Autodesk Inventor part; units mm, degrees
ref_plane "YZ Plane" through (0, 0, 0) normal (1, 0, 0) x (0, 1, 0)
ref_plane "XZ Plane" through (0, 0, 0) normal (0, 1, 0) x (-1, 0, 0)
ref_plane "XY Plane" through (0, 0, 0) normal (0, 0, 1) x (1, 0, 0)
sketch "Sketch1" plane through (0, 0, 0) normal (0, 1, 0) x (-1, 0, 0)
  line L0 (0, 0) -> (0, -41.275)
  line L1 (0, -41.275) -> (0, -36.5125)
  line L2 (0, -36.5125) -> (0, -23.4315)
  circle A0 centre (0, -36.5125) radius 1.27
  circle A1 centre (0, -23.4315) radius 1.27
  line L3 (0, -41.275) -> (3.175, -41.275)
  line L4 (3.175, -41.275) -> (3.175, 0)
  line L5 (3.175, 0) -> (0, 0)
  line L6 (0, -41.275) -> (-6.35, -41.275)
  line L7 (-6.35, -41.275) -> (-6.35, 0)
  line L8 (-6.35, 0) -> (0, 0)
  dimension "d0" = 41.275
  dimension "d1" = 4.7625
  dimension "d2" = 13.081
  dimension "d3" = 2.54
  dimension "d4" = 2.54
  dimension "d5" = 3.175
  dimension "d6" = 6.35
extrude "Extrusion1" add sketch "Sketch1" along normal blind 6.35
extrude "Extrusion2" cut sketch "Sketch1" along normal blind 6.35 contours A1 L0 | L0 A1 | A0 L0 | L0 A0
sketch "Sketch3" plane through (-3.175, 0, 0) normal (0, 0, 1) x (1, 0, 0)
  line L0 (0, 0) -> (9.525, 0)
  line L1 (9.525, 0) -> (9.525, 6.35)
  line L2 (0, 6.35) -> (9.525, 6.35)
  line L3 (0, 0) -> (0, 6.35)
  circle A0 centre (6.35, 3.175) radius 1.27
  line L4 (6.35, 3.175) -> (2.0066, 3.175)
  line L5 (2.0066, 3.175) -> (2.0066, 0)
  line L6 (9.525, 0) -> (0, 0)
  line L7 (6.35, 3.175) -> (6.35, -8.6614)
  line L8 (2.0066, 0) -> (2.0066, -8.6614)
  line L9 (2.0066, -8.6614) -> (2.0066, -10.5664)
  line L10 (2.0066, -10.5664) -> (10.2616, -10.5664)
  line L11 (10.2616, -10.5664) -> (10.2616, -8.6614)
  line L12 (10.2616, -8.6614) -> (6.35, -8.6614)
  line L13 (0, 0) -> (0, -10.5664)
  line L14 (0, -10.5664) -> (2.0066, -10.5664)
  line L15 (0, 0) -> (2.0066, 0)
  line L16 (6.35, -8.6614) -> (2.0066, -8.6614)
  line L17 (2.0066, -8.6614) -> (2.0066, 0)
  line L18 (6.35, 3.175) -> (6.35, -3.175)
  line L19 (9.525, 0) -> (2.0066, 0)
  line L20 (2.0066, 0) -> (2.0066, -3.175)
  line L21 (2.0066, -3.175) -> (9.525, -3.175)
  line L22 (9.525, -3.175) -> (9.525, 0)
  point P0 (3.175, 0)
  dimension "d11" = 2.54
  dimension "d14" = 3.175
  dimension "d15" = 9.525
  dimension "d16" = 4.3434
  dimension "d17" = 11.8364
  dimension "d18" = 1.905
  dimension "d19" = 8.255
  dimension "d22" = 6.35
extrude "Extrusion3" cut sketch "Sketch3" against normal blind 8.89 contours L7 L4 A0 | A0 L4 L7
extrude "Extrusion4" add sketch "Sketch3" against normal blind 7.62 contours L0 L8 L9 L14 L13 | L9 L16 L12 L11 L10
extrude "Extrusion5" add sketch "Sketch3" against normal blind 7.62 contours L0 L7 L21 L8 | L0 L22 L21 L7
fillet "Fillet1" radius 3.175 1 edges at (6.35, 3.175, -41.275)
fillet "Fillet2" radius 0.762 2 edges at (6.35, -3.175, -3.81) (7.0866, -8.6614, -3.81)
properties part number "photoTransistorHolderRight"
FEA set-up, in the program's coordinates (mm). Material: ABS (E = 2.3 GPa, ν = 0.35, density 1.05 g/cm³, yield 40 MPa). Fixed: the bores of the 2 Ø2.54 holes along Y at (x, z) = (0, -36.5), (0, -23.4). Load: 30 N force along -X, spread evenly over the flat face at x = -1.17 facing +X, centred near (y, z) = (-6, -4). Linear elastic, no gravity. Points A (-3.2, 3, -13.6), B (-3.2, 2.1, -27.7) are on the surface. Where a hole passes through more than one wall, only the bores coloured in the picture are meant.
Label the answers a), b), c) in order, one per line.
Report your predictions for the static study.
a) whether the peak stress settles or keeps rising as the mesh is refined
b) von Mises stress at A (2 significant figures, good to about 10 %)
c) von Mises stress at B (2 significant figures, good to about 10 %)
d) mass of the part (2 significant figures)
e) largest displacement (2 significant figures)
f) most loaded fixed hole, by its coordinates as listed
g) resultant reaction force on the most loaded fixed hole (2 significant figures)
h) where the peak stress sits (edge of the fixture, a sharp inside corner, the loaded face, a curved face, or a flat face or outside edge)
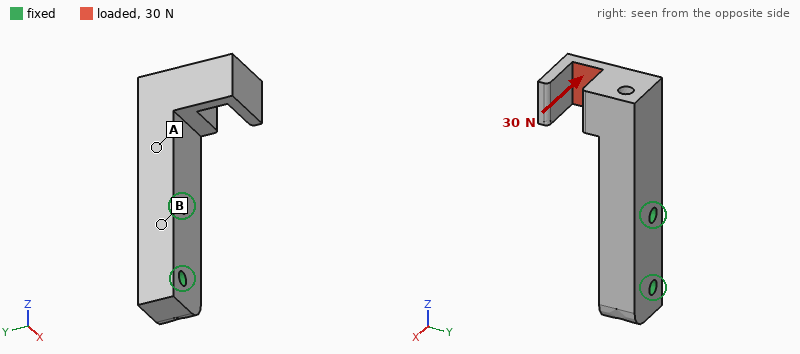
a) keeps rising
b) 5.7 MPa
c) 1.2 MPa
d) 3.0 g
e) 0.53 mm
f) (0, -23.4)
g) 64 N
h) edge of the fixture
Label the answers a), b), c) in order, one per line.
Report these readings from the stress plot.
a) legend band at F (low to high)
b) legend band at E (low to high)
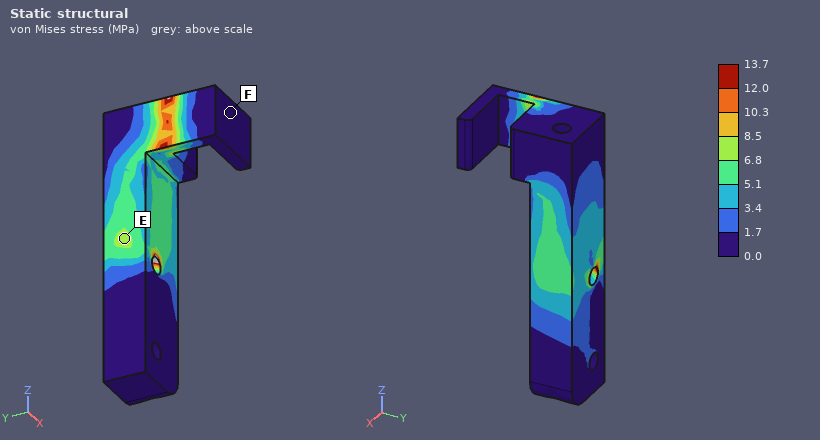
a) 0.0 to 1.7 MPa
b) 6.8 to 8.5 MPa
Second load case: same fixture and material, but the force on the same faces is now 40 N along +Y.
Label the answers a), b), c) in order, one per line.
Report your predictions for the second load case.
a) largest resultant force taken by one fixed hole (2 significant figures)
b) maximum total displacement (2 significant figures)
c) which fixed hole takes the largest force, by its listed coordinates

a) 53 N
b) 0.46 mm
c) (0, -23.4)
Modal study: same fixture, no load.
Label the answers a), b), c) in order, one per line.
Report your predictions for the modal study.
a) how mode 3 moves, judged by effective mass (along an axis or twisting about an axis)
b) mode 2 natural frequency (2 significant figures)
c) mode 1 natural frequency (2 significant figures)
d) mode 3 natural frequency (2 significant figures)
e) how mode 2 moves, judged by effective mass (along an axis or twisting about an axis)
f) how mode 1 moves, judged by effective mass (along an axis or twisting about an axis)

a) along X
b) 2000 Hz
c) 1700 Hz
d) 2800 Hz
e) along X
f) along Y
